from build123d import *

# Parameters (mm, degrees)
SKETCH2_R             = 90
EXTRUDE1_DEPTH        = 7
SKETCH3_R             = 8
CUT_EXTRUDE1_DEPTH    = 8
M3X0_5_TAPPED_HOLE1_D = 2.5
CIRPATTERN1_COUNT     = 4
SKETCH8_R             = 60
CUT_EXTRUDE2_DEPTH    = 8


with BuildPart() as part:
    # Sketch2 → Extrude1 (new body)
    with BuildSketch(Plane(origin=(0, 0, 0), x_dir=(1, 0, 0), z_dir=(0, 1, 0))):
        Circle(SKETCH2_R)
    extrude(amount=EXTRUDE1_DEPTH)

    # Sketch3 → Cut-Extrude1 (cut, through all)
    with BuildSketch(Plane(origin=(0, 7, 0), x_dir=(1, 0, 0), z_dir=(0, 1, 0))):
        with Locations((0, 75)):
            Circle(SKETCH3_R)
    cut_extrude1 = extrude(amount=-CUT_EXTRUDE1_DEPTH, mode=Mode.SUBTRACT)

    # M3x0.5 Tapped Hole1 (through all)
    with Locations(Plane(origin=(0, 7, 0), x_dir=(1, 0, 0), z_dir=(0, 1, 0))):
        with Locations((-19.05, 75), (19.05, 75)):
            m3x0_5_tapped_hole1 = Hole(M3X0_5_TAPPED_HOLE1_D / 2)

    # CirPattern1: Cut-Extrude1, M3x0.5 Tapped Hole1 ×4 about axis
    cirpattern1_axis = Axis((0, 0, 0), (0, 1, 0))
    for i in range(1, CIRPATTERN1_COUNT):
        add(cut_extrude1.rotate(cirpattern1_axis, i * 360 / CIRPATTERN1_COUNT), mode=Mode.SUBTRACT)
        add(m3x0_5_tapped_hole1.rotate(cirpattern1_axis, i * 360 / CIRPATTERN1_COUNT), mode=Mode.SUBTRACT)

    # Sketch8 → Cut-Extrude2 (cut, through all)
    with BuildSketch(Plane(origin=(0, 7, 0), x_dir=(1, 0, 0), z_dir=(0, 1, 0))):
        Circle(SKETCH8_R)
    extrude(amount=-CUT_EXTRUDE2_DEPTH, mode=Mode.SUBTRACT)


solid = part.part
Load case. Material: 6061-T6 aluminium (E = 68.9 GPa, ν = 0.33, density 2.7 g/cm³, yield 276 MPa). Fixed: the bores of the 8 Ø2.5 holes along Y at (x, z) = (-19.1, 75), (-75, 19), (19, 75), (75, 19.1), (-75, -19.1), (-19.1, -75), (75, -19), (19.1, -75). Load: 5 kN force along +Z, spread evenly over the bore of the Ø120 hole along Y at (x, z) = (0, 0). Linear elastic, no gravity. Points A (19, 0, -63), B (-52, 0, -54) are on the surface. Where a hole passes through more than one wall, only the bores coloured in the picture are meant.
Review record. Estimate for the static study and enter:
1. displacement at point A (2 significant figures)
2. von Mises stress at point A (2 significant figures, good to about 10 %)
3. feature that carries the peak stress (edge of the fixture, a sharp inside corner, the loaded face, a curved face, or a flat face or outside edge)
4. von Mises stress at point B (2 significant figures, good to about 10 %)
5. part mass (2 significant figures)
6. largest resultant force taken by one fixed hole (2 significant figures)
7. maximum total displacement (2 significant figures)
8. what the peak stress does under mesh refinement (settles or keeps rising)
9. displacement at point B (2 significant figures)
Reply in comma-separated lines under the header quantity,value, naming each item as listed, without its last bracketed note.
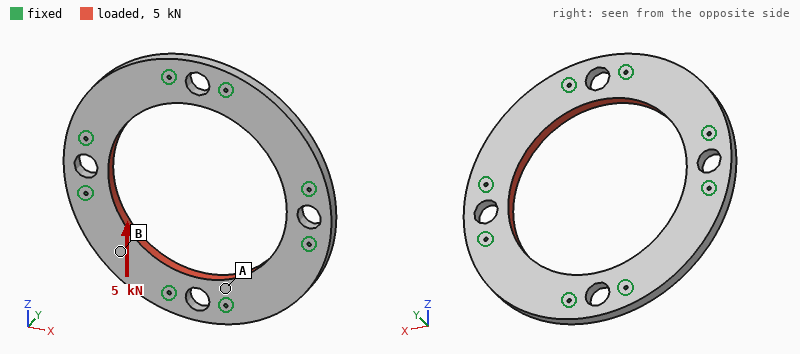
quantity,value
displacement at point A,1.1 µm
von Mises stress at point A,4.3 MPa
feature that carries the peak stress,edge of the fixture
von Mises stress at point B,1.7 MPa
part mass,250 g
largest resultant force taken by one fixed hole,660 N
maximum total displacement,3.9 µm
what the peak stress does under mesh refinement,keeps rising
displacement at point B,3.5 µm
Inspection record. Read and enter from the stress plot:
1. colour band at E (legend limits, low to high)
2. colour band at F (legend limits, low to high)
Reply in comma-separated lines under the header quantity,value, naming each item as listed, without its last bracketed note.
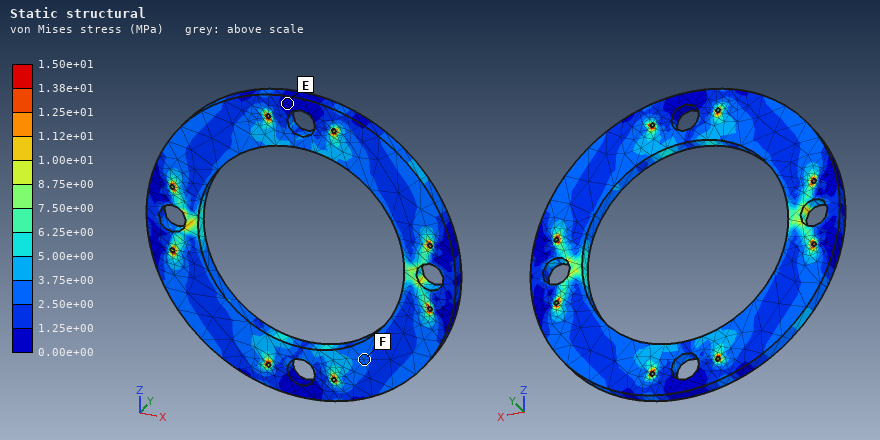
quantity,value
colour band at E,0.00e+00 to 1.25e+00 MPa
colour band at F,2.50e+00 to 3.75e+00 MPa
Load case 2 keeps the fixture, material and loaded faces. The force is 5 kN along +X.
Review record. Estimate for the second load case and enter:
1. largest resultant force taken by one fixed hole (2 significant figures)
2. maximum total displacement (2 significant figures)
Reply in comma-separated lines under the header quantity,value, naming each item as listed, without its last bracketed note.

quantity,value
largest resultant force taken by one fixed hole,660 N
maximum total displacement,3.9 µm
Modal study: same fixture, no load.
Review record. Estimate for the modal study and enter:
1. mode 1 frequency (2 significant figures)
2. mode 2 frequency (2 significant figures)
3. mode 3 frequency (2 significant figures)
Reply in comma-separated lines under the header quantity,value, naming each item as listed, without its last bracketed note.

quantity,value
mode 1 frequency,4100 Hz
mode 2 frequency,4200 Hz
mode 3 frequency,4200 Hz
